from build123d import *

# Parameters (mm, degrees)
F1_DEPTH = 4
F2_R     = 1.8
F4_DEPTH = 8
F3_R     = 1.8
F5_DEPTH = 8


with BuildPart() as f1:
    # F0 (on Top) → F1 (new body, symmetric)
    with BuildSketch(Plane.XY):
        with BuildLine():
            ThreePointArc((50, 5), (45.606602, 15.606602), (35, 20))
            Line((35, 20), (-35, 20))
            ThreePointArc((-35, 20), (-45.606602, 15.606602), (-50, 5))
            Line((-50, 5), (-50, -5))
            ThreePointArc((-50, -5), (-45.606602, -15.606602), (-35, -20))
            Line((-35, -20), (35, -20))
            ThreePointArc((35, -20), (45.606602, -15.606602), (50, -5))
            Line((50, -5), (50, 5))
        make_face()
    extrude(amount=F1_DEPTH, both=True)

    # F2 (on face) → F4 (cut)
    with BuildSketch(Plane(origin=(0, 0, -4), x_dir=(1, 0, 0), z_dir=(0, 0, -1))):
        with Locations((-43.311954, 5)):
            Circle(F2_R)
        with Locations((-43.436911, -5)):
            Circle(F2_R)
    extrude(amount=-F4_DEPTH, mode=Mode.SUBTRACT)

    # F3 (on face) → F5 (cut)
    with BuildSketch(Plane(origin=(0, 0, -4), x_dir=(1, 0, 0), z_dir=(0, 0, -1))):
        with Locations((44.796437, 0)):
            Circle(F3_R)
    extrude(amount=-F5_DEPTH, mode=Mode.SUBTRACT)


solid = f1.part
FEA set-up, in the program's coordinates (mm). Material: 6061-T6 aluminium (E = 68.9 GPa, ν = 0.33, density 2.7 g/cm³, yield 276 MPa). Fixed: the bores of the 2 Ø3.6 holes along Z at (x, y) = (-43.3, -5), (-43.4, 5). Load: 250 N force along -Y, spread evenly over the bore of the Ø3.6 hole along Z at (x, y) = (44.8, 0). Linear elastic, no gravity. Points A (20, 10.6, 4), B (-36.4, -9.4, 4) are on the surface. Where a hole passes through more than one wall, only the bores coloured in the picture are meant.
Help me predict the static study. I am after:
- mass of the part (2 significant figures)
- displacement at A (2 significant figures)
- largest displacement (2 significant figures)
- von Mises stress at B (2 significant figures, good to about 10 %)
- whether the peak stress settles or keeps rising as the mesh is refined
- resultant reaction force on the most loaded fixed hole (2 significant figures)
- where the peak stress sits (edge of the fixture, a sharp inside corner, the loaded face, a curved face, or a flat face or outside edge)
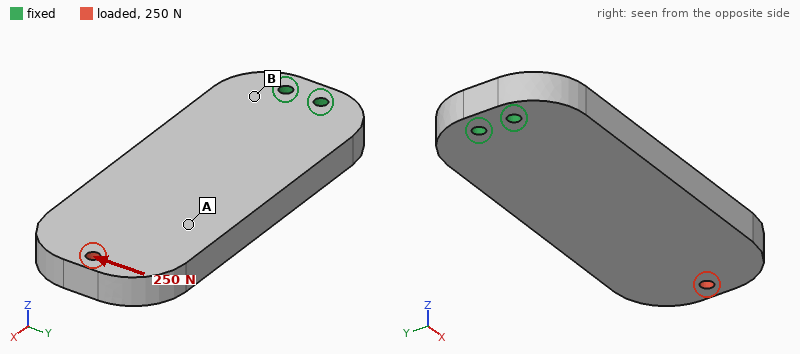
82 g
37 µm
58 µm
10 MPa
keeps rising
1.7 kN
edge of the fixture
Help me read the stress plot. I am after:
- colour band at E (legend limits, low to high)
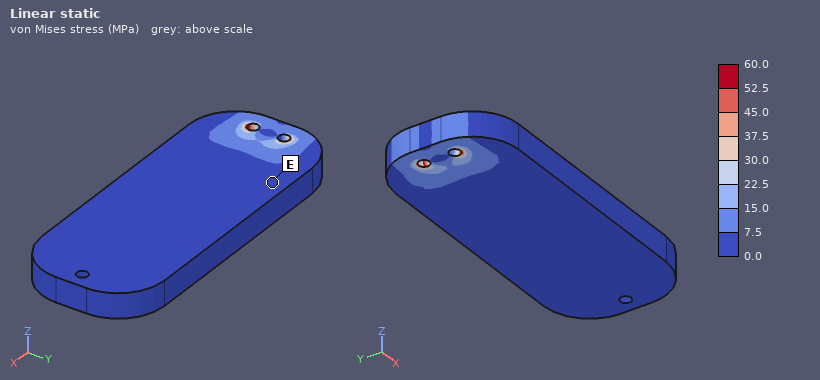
0.0 to 7.5 MPa
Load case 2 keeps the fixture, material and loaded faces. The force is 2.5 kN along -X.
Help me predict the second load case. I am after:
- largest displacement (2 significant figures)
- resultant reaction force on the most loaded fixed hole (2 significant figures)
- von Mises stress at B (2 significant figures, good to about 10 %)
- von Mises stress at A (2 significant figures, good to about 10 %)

16 µm
1.3 kN
10 MPa
8.3 MPa
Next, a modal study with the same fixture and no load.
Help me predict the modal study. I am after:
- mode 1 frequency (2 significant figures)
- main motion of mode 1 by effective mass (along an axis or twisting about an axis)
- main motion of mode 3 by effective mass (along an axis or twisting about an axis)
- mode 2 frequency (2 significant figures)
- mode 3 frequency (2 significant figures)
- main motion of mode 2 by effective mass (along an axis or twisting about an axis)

750 Hz
along Z
twisting about X
2100 Hz
3300 Hz
along Y
